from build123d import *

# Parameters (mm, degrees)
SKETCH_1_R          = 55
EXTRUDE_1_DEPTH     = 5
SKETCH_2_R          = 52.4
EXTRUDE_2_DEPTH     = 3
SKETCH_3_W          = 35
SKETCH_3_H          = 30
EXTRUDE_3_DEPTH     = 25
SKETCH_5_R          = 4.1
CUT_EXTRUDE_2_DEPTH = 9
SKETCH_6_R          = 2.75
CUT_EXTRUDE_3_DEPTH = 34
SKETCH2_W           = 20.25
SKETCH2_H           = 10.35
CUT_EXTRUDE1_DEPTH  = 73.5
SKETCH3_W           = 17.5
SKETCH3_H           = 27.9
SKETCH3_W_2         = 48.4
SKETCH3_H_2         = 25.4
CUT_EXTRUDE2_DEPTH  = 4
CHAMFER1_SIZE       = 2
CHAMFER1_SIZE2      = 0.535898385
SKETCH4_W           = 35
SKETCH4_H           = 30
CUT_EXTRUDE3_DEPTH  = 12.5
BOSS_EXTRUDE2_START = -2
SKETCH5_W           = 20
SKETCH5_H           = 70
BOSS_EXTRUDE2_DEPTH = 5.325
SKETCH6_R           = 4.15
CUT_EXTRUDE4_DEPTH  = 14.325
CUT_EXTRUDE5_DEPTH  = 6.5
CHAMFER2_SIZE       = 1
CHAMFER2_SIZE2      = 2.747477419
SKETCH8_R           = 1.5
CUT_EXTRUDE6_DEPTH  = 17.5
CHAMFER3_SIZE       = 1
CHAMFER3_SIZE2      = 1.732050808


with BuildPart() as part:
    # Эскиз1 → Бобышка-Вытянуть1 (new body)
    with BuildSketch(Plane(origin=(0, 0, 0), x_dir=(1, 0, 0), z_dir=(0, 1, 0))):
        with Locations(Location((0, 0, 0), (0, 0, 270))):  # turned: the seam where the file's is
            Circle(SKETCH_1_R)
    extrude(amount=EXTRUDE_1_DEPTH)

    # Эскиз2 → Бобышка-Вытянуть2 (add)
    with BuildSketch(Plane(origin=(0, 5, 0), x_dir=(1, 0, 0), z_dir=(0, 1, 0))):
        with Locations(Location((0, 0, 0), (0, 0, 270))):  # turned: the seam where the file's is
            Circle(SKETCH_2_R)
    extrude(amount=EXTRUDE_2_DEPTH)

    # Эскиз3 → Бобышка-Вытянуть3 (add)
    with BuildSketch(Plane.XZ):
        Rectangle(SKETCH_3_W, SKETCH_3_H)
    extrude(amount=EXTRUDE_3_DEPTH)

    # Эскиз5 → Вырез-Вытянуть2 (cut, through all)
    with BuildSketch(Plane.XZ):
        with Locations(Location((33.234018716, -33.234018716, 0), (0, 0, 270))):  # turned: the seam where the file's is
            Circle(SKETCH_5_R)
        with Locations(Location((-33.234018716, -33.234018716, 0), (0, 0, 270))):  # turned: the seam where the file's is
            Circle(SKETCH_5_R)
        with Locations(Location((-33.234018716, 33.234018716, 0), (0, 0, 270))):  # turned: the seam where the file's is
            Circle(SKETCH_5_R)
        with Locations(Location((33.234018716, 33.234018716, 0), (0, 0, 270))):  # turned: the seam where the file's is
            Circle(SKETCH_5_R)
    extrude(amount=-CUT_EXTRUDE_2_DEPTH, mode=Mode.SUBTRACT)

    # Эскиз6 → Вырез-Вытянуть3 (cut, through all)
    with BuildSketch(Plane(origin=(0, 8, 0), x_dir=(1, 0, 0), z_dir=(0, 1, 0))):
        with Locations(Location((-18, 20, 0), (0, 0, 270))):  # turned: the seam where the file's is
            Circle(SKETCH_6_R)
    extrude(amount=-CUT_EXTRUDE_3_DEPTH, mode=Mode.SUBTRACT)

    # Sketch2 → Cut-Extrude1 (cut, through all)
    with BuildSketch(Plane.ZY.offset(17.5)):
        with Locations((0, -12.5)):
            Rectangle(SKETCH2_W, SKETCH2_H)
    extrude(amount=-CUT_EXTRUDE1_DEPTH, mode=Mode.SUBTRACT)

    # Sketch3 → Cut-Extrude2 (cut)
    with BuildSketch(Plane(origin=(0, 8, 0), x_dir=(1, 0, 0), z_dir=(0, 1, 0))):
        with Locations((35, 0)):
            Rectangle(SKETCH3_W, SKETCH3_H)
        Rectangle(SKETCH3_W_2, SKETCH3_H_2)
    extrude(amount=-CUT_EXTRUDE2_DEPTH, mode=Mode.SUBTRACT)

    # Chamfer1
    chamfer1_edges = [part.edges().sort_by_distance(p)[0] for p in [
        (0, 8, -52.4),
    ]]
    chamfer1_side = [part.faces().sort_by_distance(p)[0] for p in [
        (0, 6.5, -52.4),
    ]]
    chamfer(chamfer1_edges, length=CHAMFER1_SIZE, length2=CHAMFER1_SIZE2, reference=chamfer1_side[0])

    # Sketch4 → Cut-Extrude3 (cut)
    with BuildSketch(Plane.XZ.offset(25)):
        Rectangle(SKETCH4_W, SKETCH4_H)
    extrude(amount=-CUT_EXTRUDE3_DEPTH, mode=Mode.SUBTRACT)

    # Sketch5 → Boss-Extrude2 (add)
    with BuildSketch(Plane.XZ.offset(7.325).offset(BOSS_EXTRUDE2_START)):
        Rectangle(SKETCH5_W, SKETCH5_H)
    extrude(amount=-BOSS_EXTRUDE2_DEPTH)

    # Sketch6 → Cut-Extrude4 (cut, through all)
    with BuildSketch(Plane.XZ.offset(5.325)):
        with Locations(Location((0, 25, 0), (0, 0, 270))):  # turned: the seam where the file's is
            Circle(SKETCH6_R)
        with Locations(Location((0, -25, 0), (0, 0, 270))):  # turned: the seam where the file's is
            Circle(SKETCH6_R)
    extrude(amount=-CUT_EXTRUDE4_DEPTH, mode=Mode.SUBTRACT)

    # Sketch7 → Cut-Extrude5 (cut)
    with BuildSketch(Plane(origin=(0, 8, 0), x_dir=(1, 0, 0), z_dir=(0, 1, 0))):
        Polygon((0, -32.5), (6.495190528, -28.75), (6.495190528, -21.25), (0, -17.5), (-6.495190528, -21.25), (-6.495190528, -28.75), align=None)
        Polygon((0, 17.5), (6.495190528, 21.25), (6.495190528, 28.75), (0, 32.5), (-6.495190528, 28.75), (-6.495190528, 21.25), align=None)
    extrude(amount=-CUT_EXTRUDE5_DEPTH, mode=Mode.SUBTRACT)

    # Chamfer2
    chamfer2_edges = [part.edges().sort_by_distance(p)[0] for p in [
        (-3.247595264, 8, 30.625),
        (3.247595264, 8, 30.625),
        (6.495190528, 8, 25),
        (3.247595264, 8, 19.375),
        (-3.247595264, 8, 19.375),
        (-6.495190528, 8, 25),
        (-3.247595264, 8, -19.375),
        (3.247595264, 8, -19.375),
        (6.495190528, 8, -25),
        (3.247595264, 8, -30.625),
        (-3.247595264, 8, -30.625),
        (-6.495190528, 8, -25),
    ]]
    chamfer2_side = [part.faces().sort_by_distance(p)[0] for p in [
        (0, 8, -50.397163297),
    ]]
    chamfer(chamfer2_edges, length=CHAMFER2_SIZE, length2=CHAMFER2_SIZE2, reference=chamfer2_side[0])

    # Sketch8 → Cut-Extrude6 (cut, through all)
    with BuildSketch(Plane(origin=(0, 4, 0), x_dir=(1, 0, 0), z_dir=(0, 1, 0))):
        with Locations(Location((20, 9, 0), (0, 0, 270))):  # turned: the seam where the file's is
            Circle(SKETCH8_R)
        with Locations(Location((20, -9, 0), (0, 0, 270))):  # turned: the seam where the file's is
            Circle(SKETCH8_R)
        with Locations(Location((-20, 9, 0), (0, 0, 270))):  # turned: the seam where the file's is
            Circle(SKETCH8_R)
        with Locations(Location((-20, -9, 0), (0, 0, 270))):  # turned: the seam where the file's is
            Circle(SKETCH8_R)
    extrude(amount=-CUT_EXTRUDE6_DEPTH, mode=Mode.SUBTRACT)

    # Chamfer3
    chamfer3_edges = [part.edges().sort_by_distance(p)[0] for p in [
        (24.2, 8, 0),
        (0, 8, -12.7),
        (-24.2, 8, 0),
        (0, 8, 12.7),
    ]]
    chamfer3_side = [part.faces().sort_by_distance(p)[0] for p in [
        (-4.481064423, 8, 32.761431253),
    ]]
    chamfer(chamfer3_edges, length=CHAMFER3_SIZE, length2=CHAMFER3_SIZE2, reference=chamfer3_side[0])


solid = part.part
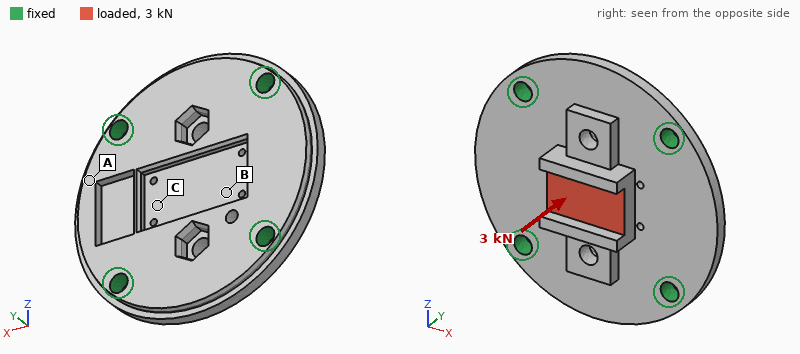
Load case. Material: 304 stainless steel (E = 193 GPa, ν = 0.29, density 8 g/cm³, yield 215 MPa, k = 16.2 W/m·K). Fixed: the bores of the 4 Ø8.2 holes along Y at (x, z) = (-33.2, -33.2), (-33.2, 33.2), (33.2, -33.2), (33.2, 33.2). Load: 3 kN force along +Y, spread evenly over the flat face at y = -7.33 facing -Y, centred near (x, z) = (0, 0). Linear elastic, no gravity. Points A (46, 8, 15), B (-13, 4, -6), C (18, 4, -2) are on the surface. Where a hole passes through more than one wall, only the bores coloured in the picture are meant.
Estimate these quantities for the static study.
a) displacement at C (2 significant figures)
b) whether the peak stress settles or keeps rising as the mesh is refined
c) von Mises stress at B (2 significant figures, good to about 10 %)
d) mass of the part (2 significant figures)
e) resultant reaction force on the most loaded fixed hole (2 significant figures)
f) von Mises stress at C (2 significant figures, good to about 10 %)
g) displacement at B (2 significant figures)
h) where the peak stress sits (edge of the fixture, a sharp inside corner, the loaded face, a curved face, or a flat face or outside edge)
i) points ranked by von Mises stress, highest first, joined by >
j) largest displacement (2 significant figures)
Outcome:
10 µm
keeps rising
11 MPa
600 g
1.2 kN
19 MPa
9.8 µm
edge of the fixture
C > B > A
10 µm
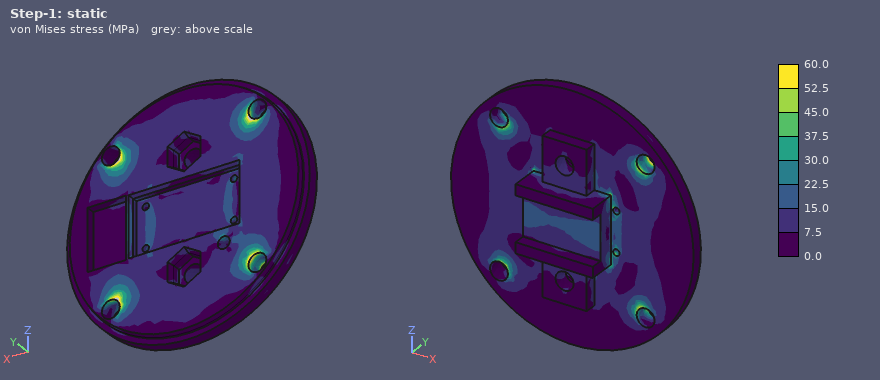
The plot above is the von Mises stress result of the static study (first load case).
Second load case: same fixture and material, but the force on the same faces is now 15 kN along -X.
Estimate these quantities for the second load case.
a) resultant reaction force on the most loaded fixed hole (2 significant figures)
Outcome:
4.6 kN
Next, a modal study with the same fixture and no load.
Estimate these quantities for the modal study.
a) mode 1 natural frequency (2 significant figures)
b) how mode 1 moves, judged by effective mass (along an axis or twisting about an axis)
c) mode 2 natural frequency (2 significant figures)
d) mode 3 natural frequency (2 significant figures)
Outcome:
6400 Hz
along Y
7800 Hz
7900 Hz
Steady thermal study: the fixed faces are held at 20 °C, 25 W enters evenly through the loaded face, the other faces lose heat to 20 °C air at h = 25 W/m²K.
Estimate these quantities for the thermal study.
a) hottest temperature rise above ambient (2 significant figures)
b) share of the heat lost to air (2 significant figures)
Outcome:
58 K
38 %
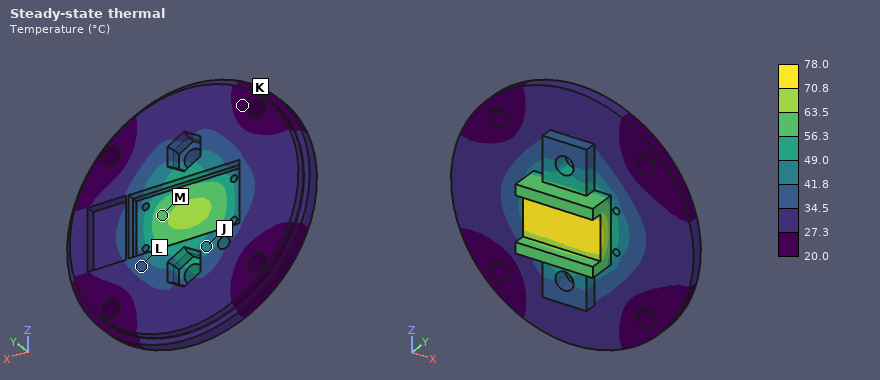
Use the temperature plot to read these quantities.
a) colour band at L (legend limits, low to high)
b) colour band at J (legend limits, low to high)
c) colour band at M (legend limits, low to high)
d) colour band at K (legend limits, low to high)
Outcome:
34.5 to 41.8 °C
41.8 to 49.0 °C
56.3 to 63.5 °C
20.0 to 27.3 °C
